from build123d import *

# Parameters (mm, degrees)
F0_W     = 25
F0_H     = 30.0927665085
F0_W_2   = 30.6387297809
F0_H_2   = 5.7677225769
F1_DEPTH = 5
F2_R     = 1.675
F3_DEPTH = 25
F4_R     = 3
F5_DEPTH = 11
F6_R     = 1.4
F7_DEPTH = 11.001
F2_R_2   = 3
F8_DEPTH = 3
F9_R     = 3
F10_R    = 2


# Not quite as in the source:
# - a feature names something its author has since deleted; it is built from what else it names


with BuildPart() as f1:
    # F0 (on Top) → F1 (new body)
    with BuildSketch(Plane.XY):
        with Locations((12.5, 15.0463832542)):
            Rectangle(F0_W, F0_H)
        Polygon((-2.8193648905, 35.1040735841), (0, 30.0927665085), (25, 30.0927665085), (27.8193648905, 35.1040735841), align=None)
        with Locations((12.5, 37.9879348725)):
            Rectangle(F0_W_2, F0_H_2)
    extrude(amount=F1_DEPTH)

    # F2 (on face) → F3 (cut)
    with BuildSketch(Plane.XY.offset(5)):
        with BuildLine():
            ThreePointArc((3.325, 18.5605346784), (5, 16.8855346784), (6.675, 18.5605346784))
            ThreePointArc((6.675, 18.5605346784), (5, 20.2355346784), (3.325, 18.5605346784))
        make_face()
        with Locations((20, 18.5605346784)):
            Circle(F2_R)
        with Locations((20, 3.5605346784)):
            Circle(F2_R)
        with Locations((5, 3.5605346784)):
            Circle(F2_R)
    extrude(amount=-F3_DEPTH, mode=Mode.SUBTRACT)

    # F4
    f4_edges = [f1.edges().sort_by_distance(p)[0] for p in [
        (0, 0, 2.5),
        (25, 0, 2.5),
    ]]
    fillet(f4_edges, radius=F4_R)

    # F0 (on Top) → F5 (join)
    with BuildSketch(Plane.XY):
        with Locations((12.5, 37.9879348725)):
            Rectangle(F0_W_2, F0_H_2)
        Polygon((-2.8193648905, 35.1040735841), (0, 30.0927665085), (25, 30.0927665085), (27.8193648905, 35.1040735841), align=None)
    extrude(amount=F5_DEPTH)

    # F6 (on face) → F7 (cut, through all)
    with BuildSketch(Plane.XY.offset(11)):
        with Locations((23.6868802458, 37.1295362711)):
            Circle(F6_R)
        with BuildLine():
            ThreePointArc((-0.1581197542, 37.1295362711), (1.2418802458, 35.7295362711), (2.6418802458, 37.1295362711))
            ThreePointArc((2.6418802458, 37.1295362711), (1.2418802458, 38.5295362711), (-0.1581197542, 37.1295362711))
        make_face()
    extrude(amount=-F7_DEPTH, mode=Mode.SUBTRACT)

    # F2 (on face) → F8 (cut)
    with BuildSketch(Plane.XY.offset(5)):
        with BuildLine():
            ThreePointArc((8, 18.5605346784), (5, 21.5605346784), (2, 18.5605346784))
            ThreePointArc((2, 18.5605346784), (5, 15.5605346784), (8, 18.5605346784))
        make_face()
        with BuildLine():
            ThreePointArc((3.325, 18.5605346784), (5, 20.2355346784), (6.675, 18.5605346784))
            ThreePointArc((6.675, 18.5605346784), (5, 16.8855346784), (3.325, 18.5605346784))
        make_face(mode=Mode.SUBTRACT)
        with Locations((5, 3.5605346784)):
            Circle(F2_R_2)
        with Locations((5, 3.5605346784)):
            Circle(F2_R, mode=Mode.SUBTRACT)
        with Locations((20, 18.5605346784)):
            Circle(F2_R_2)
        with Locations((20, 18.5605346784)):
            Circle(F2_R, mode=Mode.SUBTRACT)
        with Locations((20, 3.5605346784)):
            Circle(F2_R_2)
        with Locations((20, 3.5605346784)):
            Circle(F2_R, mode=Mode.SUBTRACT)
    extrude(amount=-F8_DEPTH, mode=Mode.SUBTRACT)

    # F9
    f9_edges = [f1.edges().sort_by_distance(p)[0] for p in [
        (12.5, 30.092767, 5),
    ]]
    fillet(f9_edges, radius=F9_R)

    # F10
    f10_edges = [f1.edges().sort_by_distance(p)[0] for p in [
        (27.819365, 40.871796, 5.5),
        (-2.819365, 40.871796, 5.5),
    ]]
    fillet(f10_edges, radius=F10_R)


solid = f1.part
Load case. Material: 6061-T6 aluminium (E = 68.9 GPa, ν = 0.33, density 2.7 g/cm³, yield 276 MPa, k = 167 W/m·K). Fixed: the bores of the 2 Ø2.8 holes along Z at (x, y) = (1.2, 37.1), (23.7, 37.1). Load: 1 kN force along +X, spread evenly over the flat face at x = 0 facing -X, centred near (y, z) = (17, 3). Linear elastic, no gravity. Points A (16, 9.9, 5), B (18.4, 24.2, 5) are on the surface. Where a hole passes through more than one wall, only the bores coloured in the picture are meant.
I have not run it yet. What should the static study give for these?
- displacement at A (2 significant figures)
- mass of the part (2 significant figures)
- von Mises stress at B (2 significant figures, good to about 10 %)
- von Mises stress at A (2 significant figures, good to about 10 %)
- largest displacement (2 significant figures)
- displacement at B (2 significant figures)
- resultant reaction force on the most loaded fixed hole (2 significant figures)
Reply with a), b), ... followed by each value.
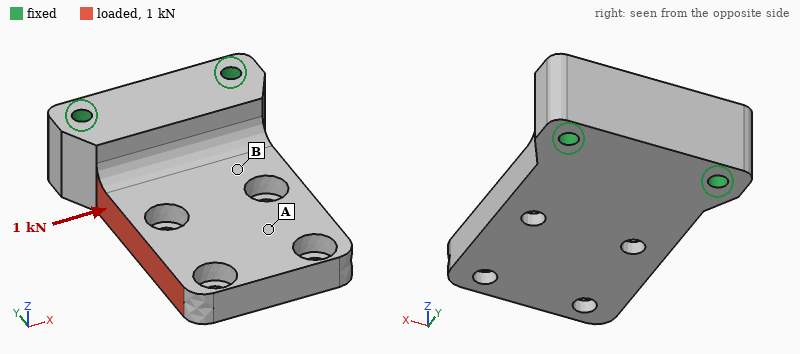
a) 15 µm
b) 18 g
c) 22 MPa
d) 4.9 MPa
e) 22 µm
f) 4.7 µm
g) 1.0 kN
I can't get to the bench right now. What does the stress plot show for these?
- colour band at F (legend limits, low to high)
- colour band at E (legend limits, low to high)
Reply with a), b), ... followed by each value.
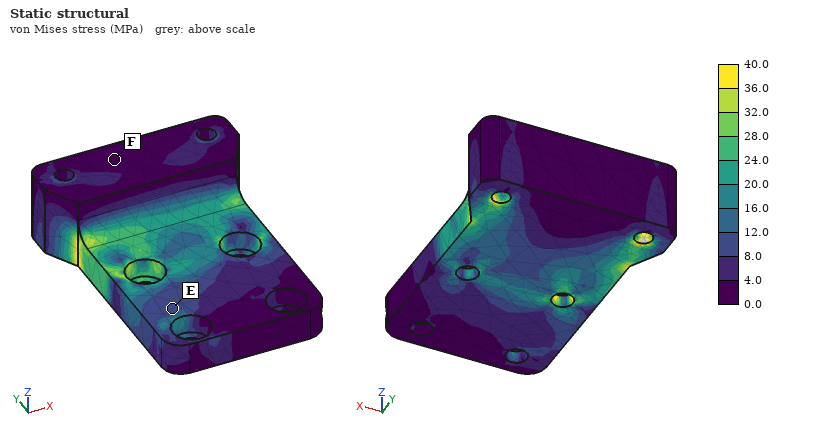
a) 0.0 to 4.0 MPa
b) 8.0 to 12.0 MPa
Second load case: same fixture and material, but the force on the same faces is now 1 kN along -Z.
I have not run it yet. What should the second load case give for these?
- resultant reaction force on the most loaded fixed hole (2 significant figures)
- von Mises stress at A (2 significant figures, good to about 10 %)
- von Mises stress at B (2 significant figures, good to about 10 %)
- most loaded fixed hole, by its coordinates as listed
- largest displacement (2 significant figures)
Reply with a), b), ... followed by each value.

a) 1.0 kN
b) 37 MPa
c) 86 MPa
d) (1.2, 37.1)
e) 0.29 mm
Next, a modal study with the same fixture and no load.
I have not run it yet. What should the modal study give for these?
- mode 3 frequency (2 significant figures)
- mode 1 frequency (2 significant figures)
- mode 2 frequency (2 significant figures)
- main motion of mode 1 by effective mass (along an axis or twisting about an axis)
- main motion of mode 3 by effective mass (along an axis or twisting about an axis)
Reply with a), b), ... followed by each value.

a) 14 kHz
b) 4100 Hz
c) 11 kHz
d) along Z
e) along X
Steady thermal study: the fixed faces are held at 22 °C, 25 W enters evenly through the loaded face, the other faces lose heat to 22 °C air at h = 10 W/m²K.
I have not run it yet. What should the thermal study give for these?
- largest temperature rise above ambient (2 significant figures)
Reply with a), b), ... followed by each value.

a) 33 K
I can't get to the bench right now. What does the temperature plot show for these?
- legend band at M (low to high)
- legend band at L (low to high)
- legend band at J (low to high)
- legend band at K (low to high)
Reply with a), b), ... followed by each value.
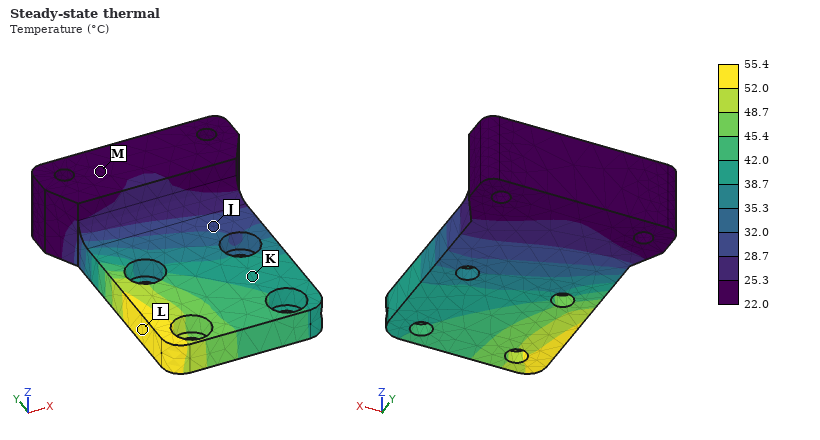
a) 22.0 to 25.3 °C
b) 52.0 to 55.4 °C
c) 28.7 to 32.0 °C
d) 38.7 to 42.0 °C
